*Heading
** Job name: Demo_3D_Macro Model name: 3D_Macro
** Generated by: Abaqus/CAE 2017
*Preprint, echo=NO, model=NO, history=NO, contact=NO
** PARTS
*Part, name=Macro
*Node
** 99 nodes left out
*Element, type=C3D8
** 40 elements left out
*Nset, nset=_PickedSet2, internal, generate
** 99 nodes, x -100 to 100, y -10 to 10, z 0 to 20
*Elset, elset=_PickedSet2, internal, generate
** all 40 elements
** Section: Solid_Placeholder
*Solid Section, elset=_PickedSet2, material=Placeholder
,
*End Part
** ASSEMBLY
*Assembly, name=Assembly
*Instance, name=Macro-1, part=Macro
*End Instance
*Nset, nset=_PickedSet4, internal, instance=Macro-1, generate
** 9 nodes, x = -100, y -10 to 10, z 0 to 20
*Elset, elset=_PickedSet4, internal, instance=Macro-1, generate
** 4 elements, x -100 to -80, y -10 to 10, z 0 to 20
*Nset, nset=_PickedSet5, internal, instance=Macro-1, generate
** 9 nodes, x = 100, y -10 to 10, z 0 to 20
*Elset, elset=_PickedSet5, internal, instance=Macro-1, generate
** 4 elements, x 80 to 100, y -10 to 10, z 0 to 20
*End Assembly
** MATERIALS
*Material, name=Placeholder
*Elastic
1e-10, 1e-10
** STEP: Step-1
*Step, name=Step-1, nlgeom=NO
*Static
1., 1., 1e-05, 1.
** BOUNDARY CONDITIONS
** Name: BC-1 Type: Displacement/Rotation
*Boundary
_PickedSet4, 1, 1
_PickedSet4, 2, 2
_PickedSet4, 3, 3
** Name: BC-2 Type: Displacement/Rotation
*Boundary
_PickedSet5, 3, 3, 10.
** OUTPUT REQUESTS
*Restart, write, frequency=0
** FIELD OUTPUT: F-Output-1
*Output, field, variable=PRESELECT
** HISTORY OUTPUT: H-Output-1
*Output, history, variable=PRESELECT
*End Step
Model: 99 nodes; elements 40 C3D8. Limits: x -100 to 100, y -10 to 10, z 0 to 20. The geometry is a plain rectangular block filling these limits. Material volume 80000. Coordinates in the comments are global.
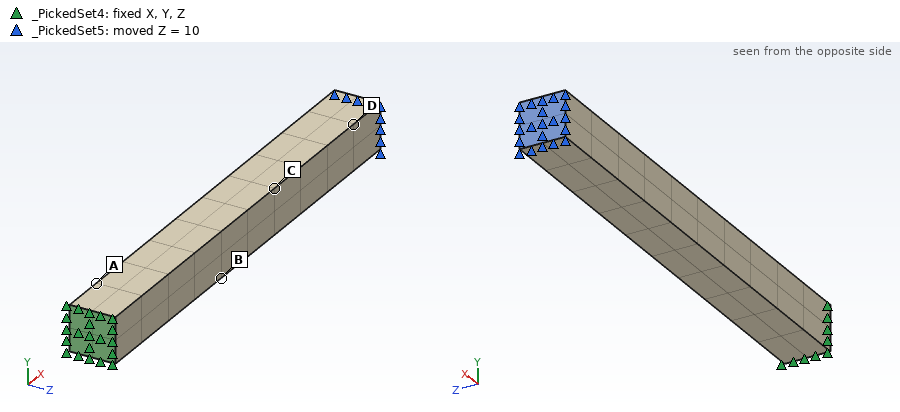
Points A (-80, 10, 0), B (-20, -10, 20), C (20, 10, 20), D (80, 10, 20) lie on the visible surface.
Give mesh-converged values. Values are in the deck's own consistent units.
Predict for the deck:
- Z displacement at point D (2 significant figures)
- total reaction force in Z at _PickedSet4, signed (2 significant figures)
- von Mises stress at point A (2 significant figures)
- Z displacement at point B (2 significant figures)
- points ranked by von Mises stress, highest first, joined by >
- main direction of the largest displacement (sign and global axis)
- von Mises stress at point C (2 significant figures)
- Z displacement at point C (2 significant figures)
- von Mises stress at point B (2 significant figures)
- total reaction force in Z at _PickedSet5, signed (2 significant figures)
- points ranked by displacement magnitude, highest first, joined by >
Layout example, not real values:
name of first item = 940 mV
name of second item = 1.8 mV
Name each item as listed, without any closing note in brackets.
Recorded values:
Z displacement at point D = 8.5
total reaction force in Z at _PickedSet4, signed = -5.0e-12
von Mises stress at point A = 6.7e-13
Z displacement at point B = 2.1
points ranked by von Mises stress, highest first, joined by > = A > B > C > D
main direction of the largest displacement = +Z
von Mises stress at point C = 3.0e-13
Z displacement at point C = 4.3
von Mises stress at point B = 4.5e-13
total reaction force in Z at _PickedSet5, signed = 5.0e-12
points ranked by displacement magnitude, highest first, joined by > = D > C > B > A
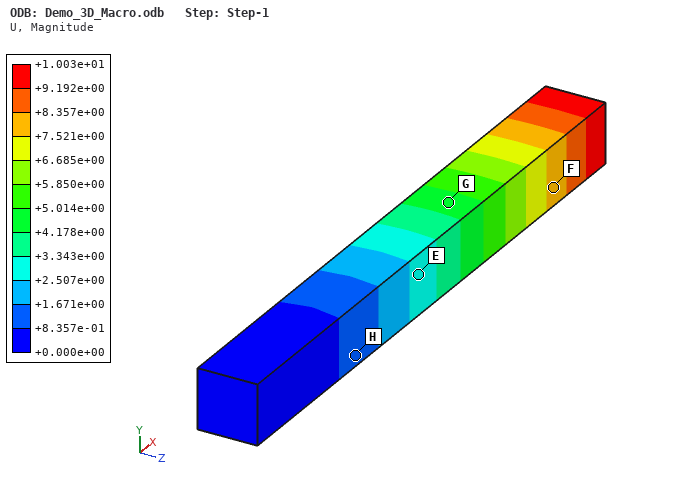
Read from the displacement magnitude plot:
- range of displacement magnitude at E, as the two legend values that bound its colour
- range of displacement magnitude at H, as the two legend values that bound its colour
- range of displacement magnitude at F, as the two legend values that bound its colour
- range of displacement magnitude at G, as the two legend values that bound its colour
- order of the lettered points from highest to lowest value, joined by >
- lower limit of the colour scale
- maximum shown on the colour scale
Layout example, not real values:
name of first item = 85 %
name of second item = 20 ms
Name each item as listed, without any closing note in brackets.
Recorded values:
range of displacement magnitude at E, as the two legend values that bound its colour = +2.507e+00 to +3.343e+00
range of displacement magnitude at H, as the two legend values that bound its colour = +8.357e-01 to +1.671e+00
range of displacement magnitude at F, as the two legend values that bound its colour = +7.521e+00 to +8.357e+00
range of displacement magnitude at G, as the two legend values that bound its colour = +4.178e+00 to +5.014e+00
order of the lettered points from highest to lowest value, joined by > = F > G > E > H
lower limit of the colour scale = +0.000e+00
maximum shown on the colour scale = +1.003e+01
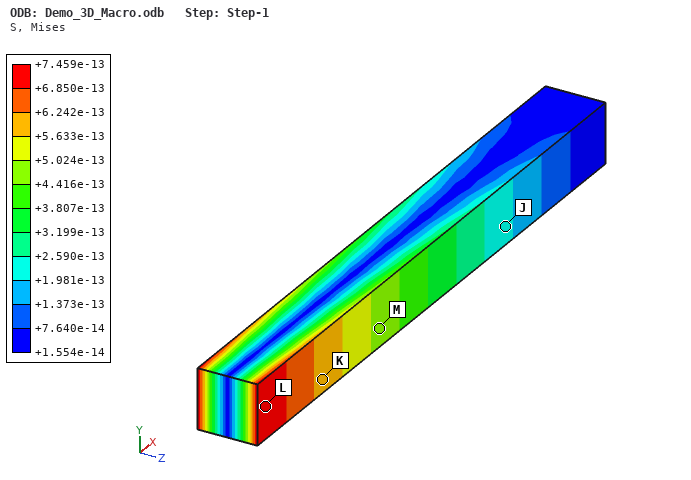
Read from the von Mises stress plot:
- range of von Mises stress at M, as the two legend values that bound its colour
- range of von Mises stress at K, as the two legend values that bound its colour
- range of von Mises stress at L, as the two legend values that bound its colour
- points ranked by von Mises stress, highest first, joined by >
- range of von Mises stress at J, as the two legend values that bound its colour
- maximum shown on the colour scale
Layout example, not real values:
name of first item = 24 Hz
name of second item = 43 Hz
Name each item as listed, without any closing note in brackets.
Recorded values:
range of von Mises stress at M, as the two legend values that bound its colour = +4.416e-13 to +5.024e-13
range of von Mises stress at K, as the two legend values that bound its colour = +5.633e-13 to +6.242e-13
range of von Mises stress at L, as the two legend values that bound its colour = +6.850e-13 to +7.459e-13
points ranked by von Mises stress, highest first, joined by > = L > K > M > J
range of von Mises stress at J, as the two legend values that bound its colour = +1.981e-13 to +2.590e-13
maximum shown on the colour scale = +7.459e-13
